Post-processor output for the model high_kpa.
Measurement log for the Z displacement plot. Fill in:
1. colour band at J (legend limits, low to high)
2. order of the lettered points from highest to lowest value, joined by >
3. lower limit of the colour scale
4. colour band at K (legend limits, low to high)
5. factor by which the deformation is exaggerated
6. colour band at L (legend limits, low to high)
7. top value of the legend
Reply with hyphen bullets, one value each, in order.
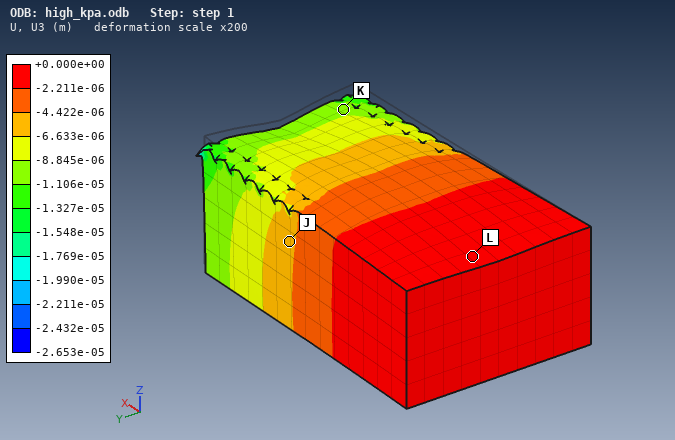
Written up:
- -6.633e-06 to -4.422e-06 m
- L > J > K
- -2.653e-05 m
- -1.106e-05 to -8.845e-06 m
- 200
- -2.211e-06 to +0.000e+00 m
- +0.000e+00 m
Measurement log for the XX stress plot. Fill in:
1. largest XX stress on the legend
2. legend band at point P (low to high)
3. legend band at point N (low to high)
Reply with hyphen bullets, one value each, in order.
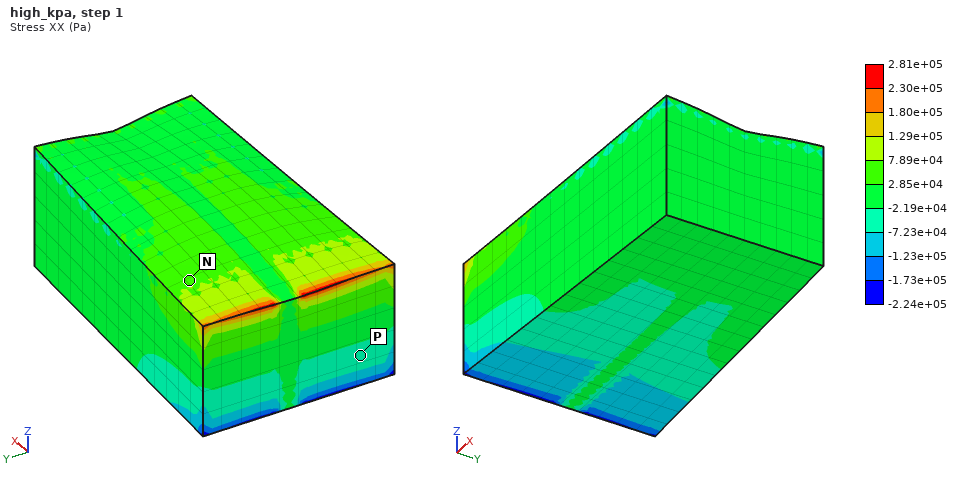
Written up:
- 2.81e+05 Pa
- -7.23e+04 to -2.19e+04 Pa
- 2.85e+04 to 7.89e+04 Pa
